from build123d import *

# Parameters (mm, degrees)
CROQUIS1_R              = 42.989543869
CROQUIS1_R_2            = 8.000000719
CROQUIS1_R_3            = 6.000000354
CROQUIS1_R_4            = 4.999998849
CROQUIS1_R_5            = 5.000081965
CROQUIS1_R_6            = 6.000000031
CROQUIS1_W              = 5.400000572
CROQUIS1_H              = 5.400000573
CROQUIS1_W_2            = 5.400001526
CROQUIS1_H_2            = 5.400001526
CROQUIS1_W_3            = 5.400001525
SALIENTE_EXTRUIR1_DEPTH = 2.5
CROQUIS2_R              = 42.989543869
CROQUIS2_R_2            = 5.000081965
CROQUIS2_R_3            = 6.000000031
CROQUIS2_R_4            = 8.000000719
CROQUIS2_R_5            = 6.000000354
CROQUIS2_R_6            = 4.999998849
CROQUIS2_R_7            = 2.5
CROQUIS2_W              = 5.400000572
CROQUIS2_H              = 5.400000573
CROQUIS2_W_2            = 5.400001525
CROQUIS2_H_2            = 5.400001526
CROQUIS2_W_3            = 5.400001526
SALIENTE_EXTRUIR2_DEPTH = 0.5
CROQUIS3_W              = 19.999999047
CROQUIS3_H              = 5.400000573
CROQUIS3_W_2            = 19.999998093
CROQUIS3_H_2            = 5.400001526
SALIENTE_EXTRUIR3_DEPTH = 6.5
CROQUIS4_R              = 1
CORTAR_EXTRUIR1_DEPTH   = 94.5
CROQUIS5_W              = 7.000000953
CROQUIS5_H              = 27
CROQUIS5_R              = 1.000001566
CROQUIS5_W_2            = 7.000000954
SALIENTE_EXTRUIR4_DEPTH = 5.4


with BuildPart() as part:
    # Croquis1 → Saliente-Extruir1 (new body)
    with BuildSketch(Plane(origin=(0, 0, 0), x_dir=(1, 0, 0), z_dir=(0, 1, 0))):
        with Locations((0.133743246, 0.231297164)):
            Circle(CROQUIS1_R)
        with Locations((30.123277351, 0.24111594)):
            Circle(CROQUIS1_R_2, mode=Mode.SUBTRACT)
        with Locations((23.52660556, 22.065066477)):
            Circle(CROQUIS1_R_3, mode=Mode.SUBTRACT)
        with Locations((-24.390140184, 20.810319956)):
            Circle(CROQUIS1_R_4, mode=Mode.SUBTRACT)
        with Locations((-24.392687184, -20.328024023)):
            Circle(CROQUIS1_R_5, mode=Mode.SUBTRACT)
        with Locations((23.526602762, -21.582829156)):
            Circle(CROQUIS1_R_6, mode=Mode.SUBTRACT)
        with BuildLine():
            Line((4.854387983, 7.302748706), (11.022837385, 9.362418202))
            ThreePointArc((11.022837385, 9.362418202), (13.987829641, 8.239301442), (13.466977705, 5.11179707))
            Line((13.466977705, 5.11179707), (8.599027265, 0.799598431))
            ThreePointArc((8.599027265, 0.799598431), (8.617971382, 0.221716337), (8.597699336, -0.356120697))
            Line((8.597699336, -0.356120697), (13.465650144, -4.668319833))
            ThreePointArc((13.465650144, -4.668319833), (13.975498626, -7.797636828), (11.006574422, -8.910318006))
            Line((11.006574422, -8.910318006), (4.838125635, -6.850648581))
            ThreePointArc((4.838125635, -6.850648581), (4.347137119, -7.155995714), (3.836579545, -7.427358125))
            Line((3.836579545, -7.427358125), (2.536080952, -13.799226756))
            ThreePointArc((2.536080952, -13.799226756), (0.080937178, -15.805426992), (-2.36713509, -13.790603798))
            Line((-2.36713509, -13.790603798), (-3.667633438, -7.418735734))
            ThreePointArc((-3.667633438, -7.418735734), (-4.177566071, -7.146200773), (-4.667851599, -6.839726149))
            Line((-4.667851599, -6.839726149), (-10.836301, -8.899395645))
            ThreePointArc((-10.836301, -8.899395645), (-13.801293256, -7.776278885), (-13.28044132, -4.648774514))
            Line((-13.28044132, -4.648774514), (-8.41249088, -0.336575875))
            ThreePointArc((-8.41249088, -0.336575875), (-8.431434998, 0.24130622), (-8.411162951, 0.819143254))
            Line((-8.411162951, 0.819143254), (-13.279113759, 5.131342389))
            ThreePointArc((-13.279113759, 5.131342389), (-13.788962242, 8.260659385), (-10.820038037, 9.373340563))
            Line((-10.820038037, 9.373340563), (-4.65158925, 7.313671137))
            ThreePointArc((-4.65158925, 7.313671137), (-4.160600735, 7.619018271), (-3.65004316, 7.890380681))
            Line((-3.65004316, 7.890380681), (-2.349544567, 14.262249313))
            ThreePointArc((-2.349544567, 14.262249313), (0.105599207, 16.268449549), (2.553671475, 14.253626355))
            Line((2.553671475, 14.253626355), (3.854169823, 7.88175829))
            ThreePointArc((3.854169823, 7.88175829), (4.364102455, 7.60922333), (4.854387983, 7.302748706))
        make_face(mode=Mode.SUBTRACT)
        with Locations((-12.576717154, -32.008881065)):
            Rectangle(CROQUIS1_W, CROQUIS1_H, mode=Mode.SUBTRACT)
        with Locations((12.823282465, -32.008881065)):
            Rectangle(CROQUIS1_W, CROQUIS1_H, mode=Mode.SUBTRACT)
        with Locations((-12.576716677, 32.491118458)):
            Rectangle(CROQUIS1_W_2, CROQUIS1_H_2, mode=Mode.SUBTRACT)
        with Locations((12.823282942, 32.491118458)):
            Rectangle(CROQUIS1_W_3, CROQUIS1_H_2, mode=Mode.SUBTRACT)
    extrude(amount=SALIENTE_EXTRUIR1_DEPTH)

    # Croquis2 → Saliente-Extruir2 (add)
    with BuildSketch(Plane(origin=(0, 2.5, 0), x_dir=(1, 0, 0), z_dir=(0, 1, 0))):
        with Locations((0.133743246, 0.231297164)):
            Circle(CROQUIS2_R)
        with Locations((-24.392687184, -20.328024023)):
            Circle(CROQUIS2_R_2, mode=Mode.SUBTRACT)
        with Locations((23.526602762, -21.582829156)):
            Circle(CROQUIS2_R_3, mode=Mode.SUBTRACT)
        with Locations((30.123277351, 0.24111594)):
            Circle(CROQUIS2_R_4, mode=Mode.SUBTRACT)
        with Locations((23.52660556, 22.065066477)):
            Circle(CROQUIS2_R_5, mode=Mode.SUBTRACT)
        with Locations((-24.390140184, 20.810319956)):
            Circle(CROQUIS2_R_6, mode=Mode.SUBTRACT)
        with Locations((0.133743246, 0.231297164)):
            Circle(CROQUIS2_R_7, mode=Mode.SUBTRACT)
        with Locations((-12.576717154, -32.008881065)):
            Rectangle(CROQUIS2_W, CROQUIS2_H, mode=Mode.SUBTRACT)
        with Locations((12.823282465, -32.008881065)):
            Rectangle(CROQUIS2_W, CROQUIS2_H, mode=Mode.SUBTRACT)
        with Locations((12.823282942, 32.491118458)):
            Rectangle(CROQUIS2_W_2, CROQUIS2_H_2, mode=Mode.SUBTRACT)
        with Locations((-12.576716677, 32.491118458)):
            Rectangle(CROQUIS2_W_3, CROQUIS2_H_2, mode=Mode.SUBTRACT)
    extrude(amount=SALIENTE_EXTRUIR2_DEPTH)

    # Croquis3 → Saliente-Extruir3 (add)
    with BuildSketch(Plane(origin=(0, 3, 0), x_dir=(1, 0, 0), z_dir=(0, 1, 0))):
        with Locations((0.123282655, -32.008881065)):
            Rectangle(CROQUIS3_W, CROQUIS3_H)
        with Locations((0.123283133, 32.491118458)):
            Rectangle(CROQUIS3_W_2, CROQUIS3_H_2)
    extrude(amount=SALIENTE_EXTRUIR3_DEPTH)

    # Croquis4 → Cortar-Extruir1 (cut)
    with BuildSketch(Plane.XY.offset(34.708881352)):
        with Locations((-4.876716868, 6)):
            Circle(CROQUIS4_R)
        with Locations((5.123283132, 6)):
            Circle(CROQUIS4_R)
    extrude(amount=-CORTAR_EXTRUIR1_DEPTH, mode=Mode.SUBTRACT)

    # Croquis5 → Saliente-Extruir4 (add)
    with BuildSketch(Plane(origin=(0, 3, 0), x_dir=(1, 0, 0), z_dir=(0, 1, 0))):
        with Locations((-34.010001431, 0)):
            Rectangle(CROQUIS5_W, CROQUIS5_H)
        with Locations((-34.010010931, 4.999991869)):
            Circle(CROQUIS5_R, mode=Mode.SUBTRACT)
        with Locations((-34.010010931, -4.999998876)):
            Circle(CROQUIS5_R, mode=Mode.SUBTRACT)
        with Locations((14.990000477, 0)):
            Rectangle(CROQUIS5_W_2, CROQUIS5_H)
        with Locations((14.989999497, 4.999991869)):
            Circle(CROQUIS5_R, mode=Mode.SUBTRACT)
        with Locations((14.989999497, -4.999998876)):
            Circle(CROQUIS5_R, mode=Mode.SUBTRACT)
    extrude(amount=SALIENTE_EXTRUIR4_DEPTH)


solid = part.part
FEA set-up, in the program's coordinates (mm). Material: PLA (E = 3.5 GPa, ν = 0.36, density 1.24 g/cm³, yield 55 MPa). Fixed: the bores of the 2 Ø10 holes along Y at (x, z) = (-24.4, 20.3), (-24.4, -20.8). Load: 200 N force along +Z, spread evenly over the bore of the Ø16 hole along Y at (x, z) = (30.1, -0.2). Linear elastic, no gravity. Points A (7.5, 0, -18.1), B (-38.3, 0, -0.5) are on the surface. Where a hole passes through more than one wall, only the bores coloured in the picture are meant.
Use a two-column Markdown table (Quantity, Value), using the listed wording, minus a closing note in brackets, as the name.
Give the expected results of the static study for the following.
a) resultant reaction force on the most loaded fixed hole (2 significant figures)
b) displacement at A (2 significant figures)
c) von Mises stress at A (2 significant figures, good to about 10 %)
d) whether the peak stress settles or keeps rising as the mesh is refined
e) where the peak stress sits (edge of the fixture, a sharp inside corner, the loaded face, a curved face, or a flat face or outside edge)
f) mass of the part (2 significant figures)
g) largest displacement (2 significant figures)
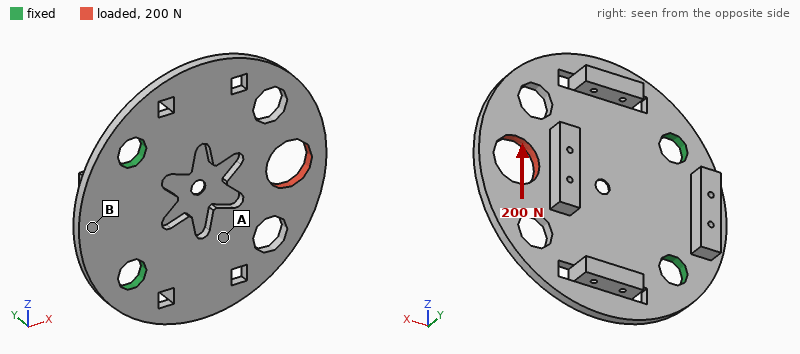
| Quantity | Value |
|---|---|
| resultant reaction force on the most loaded fixed hole | 220 N |
| displacement at A | 0.095 mm |
| von Mises stress at A | 2.8 MPa |
| whether the peak stress settles or keeps rising as the mesh is refined | keeps rising |
| where the peak stress sits | a sharp inside corner |
| mass of the part | 22 g |
| largest displacement | 0.20 mm |
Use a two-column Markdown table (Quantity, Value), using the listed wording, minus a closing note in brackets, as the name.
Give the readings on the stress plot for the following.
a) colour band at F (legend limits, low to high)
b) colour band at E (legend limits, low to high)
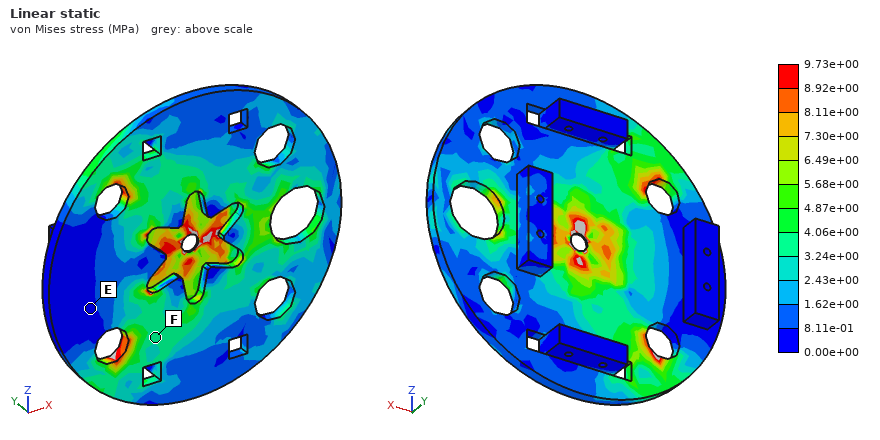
| Quantity | Value |
|---|---|
| colour band at F | 3.24e+00 to 4.06e+00 MPa |
| colour band at E | 0.00e+00 to 8.11e-01 MPa |
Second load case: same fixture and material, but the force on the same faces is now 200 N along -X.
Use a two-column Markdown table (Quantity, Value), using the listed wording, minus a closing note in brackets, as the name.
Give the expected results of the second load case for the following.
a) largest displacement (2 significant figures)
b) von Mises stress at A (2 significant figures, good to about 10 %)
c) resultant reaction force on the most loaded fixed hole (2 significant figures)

| Quantity | Value |
|---|---|
| largest displacement | 0.16 mm |
| von Mises stress at A | 2.8 MPa |
| resultant reaction force on the most loaded fixed hole | 100 N |
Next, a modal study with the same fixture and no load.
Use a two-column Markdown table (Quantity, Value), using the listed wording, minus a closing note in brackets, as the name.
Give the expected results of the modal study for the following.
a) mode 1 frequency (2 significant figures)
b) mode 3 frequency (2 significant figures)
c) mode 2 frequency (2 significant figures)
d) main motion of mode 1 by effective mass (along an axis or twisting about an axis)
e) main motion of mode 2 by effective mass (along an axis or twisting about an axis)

| Quantity | Value |
|---|---|
| mode 1 frequency | 240 Hz |
| mode 3 frequency | 1000 Hz |
| mode 2 frequency | 510 Hz |
| main motion of mode 1 by effective mass | along Y |
| main motion of mode 2 by effective mass | twisting about X |
